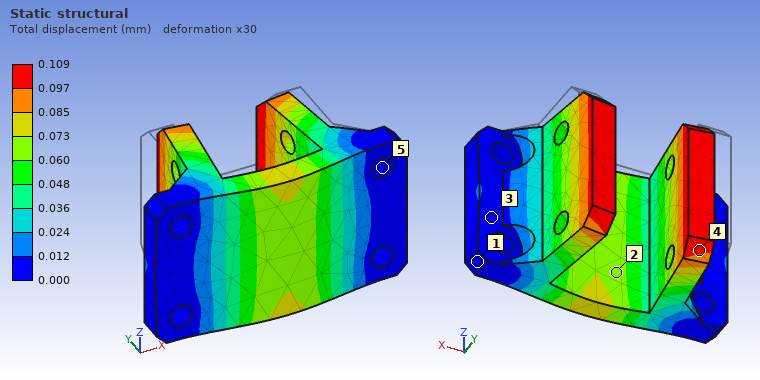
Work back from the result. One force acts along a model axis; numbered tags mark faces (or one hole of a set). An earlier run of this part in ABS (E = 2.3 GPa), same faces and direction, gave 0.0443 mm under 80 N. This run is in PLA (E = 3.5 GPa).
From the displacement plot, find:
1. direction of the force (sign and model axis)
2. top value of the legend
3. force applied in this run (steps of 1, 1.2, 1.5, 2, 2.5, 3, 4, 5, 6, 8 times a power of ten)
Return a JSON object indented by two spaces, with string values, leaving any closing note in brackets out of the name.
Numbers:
{
  "direction of the force": "-Y",
  "top value of the legend": "0.109 mm",
  "force applied in this run": "300 N"
}
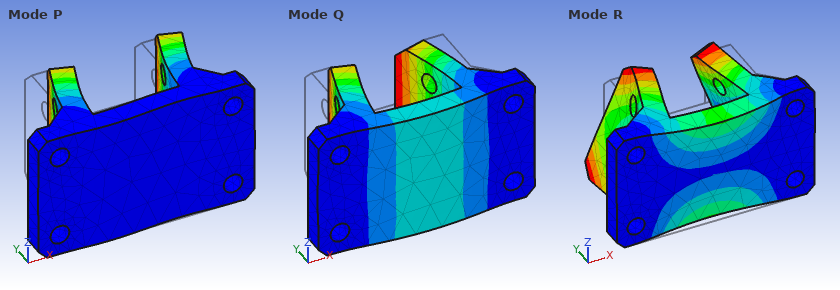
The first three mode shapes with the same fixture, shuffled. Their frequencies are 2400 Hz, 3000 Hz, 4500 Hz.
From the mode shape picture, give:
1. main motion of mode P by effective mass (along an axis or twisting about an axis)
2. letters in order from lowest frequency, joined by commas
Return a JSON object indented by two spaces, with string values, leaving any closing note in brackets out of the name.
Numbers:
{
  "main motion of mode P by effective mass": "along X",
  "letters in order from lowest frequency, joined by commas": "Q, P, R"
}
